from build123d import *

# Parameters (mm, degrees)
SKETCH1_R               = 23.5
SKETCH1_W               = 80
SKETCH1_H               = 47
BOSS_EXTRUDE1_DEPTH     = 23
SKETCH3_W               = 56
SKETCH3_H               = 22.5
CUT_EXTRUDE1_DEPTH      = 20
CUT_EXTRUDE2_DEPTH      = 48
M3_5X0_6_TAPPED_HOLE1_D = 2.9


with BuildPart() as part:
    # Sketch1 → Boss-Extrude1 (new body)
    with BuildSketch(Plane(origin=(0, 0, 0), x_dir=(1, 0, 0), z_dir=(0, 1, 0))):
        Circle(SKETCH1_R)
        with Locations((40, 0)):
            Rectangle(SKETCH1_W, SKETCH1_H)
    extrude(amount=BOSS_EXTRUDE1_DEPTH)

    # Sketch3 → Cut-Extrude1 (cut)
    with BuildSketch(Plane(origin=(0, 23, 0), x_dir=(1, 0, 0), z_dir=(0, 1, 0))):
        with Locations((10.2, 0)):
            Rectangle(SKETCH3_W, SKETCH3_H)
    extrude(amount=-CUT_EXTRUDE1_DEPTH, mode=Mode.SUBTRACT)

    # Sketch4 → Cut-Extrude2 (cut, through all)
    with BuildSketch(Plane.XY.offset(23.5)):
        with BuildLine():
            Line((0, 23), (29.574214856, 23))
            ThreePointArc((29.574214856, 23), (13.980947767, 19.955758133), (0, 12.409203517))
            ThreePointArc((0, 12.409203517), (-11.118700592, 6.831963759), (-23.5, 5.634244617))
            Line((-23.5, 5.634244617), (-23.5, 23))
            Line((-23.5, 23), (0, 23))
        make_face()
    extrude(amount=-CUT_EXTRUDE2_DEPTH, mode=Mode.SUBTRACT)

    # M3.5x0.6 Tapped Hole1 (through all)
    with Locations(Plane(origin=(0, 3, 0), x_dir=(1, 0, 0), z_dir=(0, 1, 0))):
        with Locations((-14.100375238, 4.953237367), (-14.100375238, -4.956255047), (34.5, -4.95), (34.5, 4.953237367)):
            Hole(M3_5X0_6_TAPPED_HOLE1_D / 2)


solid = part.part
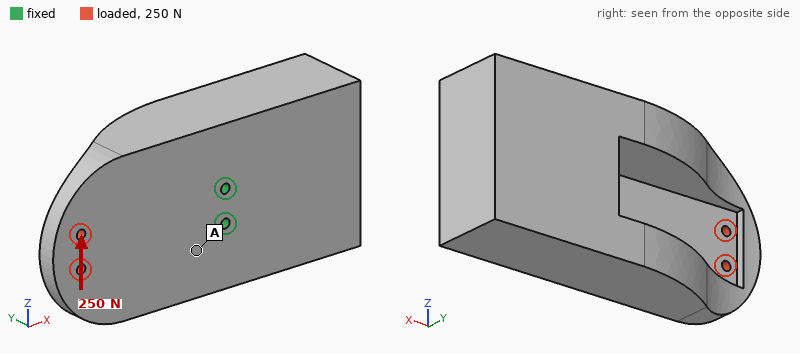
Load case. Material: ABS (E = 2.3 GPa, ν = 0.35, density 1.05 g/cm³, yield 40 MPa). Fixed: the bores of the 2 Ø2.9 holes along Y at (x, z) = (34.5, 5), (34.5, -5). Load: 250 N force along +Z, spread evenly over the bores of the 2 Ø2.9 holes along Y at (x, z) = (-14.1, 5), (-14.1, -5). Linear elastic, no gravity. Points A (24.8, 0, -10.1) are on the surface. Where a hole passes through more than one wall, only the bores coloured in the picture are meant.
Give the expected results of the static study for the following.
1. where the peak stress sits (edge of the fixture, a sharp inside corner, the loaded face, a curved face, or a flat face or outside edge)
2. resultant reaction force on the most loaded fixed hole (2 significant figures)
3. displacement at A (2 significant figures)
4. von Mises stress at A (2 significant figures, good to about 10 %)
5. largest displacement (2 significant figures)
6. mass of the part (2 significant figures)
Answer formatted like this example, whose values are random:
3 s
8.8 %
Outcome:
edge of the fixture
1.0 kN
0.23 mm
4.8 MPa
1.1 mm
75 g
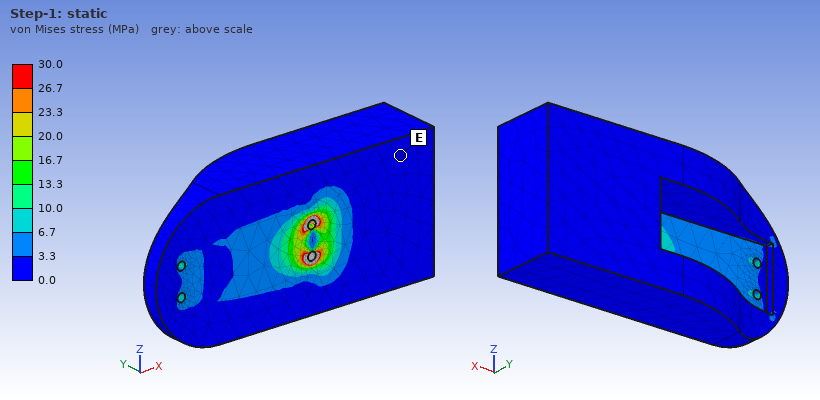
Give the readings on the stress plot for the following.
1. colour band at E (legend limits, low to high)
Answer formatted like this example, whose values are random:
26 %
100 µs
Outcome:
0.0 to 3.3 MPa
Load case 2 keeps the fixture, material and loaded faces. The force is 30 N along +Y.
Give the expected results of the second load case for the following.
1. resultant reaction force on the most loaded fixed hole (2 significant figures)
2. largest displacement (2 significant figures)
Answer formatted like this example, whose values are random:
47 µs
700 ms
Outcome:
17 N
1.3 mm
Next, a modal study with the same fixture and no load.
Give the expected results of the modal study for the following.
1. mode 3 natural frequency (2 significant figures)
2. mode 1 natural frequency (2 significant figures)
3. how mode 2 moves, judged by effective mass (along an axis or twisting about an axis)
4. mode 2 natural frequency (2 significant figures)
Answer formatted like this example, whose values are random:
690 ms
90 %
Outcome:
560 Hz
170 Hz
along Z
500 Hz
